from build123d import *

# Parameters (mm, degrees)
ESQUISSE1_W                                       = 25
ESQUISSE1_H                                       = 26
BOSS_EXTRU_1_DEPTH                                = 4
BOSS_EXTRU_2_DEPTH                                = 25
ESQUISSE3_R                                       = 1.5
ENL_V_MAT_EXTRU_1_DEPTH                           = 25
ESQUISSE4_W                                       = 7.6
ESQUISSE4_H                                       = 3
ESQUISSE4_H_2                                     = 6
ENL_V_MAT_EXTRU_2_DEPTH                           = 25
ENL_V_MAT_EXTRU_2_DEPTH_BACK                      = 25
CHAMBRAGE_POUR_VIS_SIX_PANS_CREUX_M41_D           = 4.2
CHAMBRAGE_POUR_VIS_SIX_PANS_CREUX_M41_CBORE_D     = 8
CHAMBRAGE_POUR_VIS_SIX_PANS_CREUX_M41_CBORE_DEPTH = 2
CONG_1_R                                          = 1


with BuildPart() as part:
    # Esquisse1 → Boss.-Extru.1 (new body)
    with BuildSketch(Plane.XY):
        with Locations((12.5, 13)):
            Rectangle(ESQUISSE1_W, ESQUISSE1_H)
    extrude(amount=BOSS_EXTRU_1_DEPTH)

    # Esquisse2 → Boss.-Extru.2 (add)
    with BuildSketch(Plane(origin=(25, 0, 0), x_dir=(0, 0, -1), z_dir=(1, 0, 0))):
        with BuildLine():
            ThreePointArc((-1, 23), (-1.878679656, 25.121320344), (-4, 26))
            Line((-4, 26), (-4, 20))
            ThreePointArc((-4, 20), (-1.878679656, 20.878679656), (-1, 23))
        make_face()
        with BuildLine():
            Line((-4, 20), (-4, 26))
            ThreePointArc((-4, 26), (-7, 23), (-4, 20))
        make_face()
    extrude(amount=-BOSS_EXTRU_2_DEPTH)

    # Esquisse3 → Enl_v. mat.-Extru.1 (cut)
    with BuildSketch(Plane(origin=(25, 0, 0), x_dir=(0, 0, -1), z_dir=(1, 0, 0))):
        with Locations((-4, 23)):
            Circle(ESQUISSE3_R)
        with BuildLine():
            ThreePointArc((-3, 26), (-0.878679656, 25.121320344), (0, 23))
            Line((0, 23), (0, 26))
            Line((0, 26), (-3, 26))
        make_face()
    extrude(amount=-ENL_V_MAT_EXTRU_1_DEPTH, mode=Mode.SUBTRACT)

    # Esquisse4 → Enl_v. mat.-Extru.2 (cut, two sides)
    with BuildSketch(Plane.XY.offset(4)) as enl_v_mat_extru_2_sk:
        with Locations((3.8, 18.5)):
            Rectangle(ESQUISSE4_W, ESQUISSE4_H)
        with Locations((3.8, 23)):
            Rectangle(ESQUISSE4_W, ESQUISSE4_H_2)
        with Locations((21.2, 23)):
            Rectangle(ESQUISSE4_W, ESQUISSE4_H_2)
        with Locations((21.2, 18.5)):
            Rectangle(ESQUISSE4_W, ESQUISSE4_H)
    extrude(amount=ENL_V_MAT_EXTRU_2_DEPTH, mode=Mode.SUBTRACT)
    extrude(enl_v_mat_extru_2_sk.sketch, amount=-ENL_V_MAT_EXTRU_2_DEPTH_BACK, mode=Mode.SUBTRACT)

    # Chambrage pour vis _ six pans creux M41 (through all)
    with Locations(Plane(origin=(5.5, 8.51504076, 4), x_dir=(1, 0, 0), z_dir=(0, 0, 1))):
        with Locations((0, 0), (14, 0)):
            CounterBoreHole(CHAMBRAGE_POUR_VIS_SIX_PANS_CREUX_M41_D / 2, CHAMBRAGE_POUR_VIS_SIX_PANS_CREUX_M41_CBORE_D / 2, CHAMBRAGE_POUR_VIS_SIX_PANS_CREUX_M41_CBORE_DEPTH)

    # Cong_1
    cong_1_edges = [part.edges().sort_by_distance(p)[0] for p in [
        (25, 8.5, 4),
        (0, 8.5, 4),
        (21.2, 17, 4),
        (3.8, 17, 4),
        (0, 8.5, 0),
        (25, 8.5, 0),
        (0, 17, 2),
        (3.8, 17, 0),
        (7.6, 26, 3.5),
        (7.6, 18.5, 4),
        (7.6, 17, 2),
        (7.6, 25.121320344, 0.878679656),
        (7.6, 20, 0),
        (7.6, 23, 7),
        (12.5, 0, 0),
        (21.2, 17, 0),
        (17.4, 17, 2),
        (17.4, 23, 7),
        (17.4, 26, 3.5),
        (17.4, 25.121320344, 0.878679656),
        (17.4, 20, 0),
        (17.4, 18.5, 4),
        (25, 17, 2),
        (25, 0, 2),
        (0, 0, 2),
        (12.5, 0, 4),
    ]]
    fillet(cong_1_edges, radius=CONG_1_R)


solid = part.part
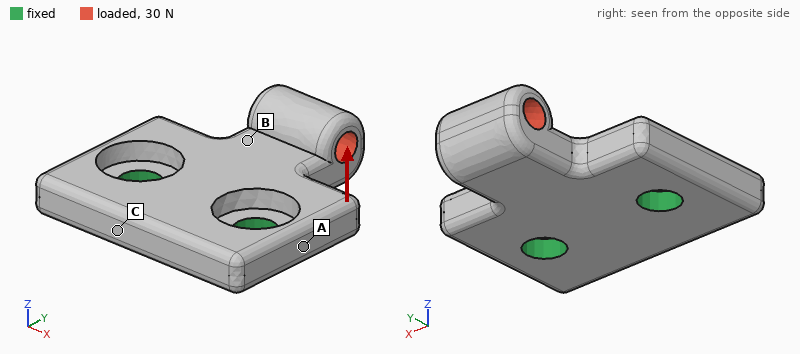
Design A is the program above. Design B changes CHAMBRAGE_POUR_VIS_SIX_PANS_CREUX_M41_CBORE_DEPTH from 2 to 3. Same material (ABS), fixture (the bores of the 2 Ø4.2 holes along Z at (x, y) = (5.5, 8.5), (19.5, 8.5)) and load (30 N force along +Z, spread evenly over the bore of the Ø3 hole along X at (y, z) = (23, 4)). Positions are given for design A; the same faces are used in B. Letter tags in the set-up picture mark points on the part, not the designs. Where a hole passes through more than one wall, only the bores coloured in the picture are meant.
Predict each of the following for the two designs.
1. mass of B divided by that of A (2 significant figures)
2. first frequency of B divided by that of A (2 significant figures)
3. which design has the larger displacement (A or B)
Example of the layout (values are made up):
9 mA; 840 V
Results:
0.96; 0.69; B
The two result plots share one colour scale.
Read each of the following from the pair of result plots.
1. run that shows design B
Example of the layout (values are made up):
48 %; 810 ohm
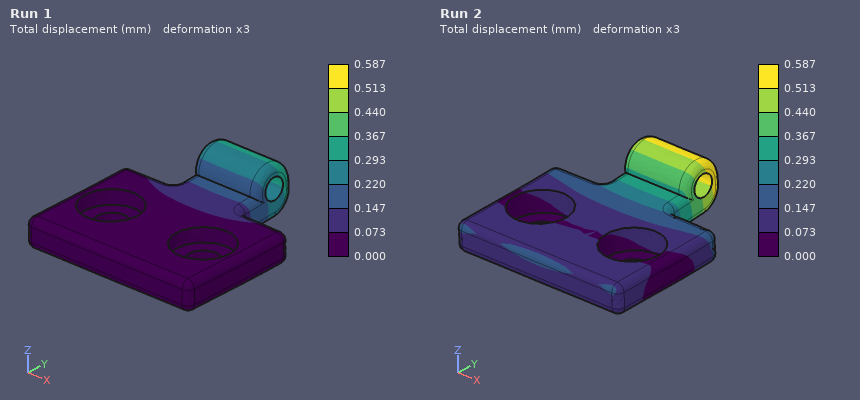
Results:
Run 2
